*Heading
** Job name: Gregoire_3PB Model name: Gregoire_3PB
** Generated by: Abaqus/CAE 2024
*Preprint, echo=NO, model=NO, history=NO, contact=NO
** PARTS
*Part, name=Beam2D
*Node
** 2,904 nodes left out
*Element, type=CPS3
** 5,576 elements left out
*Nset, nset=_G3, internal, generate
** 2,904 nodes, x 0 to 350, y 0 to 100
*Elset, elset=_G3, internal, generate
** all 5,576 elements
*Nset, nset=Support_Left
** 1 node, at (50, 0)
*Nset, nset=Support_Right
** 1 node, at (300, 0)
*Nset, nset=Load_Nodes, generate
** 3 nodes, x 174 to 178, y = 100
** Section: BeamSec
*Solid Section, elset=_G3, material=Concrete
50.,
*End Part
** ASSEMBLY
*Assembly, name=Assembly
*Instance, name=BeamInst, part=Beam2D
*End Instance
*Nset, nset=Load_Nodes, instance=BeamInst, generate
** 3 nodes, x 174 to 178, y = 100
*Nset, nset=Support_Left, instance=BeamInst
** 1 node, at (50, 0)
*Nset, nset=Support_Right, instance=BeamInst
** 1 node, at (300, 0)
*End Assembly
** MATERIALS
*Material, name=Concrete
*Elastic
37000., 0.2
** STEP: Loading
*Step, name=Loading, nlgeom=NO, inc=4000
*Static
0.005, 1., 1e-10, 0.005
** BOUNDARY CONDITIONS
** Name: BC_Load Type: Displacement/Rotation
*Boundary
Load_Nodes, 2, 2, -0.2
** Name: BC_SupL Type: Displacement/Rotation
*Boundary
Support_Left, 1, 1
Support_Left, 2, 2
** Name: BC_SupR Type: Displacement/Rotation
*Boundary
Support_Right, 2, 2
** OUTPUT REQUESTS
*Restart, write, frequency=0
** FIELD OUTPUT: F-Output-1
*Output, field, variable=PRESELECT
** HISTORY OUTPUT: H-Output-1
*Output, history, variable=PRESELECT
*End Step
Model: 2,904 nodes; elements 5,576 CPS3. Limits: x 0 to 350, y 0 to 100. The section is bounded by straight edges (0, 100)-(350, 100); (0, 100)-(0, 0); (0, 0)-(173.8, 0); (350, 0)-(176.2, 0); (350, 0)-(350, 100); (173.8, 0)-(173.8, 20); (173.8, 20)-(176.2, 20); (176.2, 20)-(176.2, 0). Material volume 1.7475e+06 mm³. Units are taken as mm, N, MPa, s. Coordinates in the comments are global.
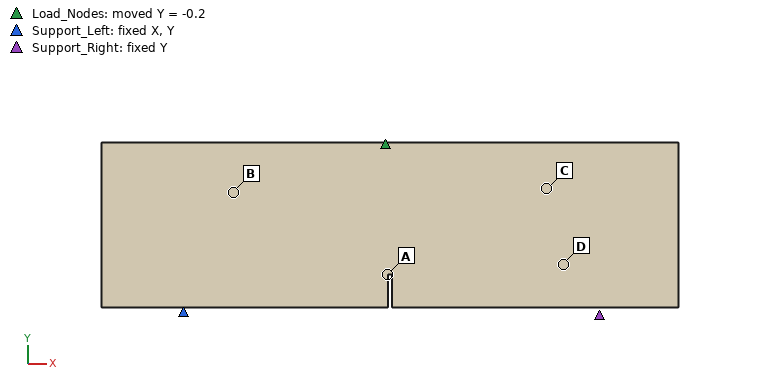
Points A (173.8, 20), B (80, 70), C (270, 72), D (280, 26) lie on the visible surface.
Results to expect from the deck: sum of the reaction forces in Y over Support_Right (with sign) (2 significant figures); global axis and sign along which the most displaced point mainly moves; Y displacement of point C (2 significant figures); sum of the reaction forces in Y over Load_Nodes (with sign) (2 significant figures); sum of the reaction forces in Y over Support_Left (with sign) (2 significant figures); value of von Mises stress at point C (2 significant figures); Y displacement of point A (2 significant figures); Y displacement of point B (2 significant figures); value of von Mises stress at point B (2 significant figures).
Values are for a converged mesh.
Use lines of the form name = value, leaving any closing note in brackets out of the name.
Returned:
sum of the reaction forces in Y over Support_Right (with sign) = 18000 N
global axis and sign along which the most displaced point mainly moves = -Y
Y displacement of point C = -0.071 mm
sum of the reaction forces in Y over Load_Nodes (with sign) = -36000 N
sum of the reaction forces in Y over Support_Left (with sign) = 18000 N
value of von Mises stress at point C = 7.6 MPa
Y displacement of point A = -0.17 mm
Y displacement of point B = -0.070 mm
value of von Mises stress at point B = 7.7 MPa
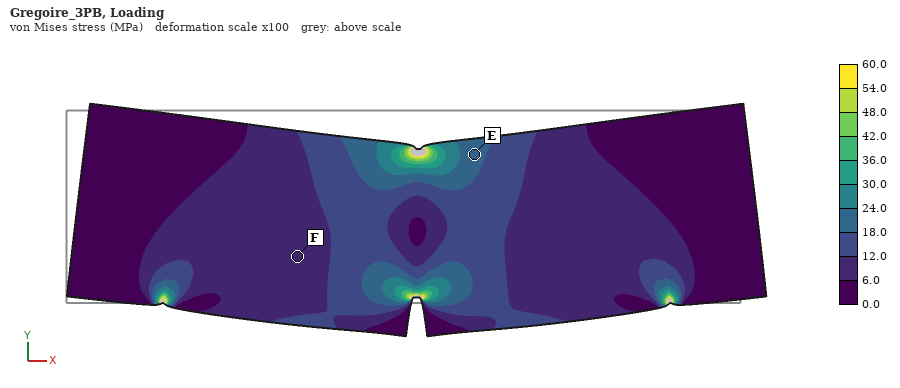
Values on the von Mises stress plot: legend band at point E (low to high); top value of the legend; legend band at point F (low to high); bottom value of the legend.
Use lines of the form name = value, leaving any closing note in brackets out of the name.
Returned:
legend band at point E = 18.0 to 24.0 MPa
top value of the legend = 60.0 MPa
legend band at point F = 6.0 to 12.0 MPa
bottom value of the legend = 0.0 MPa
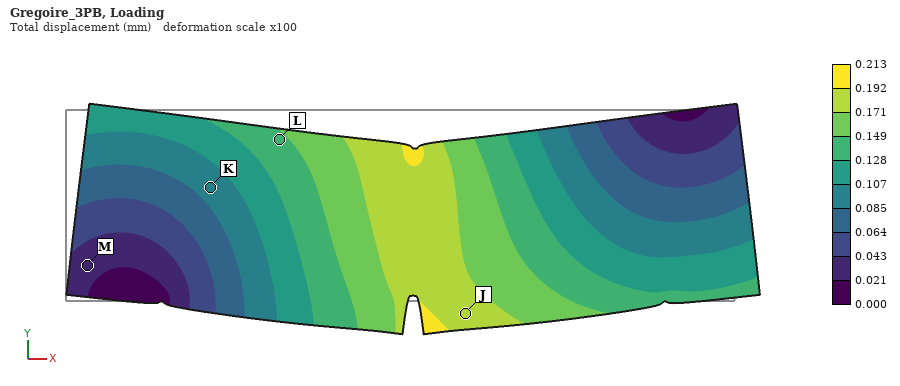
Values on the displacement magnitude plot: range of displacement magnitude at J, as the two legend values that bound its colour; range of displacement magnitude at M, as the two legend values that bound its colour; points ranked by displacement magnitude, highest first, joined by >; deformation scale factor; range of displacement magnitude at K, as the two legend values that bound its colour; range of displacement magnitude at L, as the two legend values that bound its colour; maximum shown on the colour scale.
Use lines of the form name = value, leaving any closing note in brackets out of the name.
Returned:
range of displacement magnitude at J, as the two legend values that bound its colour = 0.171 to 0.192 mm
range of displacement magnitude at M, as the two legend values that bound its colour = 0.021 to 0.043 mm
points ranked by displacement magnitude, highest first, joined by > = J > L > K > M
deformation scale factor = 100
range of displacement magnitude at K, as the two legend values that bound its colour = 0.085 to 0.107 mm
range of displacement magnitude at L, as the two legend values that bound its colour = 0.128 to 0.149 mm
maximum shown on the colour scale = 0.213 mm
